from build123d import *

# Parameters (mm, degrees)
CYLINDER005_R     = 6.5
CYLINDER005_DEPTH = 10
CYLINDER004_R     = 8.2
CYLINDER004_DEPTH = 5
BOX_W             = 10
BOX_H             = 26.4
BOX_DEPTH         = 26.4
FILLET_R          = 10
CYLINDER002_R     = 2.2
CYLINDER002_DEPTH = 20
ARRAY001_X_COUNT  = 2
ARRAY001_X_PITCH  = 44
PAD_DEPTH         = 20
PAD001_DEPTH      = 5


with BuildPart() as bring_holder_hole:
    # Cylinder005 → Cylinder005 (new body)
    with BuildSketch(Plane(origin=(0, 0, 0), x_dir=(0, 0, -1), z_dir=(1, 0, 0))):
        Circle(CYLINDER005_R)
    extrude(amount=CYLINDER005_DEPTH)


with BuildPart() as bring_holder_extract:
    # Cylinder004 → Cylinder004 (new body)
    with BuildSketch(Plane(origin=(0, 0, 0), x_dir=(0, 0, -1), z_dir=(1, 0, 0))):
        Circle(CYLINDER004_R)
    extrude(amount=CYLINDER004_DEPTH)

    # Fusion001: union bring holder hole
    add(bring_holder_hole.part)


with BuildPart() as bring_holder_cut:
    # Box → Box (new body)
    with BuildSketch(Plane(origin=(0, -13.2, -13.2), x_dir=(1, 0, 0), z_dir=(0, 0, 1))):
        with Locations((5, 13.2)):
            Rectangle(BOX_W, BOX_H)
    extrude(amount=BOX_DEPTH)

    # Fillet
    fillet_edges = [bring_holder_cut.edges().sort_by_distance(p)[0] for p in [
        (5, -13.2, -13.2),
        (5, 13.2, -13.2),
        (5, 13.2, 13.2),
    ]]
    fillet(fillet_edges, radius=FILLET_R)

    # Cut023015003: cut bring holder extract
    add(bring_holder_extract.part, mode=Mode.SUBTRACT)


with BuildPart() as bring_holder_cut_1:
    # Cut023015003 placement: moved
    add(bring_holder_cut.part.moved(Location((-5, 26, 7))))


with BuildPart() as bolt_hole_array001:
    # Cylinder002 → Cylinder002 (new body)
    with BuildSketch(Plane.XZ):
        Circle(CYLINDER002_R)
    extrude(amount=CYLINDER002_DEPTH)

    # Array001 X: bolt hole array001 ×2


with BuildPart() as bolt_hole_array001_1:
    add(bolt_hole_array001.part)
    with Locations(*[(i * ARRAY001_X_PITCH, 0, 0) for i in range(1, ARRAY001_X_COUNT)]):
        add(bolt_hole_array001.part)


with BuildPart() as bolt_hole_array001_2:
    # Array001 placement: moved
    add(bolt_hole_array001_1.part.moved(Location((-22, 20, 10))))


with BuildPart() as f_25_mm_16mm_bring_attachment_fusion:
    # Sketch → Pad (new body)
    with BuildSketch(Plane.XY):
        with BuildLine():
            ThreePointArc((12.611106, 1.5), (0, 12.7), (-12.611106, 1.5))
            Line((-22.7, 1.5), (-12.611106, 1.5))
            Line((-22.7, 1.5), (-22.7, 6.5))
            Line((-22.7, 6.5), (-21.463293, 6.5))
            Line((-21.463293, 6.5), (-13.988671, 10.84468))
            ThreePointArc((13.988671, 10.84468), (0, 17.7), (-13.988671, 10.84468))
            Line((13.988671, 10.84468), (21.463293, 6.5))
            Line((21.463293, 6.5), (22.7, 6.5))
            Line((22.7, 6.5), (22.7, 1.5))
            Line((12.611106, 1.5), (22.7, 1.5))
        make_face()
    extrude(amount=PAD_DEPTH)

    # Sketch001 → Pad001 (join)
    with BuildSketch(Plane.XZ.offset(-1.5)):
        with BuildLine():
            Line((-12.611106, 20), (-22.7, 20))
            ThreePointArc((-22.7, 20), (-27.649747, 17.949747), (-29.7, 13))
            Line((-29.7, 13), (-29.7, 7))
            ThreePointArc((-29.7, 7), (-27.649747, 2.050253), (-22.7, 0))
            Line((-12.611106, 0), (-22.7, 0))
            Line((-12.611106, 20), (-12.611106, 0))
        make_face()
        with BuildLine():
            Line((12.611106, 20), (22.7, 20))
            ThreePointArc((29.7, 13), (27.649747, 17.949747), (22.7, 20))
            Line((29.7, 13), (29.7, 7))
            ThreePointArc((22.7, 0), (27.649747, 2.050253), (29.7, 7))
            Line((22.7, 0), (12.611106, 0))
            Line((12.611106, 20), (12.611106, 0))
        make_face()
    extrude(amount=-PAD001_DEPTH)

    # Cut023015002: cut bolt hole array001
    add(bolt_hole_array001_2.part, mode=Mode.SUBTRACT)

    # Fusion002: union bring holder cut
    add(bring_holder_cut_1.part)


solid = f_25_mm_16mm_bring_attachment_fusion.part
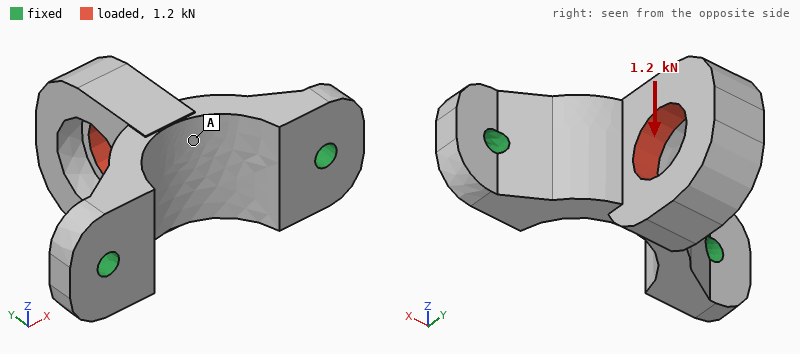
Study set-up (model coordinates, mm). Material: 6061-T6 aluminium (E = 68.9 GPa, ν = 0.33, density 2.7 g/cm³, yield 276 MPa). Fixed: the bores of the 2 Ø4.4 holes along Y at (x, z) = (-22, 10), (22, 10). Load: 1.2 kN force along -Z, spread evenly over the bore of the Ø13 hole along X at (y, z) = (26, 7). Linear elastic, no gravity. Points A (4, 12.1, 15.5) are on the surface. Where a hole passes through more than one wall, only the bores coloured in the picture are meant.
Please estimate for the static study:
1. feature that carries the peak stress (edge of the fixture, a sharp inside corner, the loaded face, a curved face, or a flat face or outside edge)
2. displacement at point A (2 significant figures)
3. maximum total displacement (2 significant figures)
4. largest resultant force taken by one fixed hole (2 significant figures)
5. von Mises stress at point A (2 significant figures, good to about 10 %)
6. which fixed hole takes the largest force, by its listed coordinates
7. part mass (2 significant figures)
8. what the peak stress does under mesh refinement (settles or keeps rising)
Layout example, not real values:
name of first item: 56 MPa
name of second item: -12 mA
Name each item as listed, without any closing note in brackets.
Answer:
feature that carries the peak stress: edge of the fixture
displacement at point A: 0.045 mm
maximum total displacement: 0.19 mm
largest resultant force taken by one fixed hole: 670 N
von Mises stress at point A: 30 MPa
which fixed hole takes the largest force, by its listed coordinates: (22, 10)
part mass: 29 g
what the peak stress does under mesh refinement: keeps rising
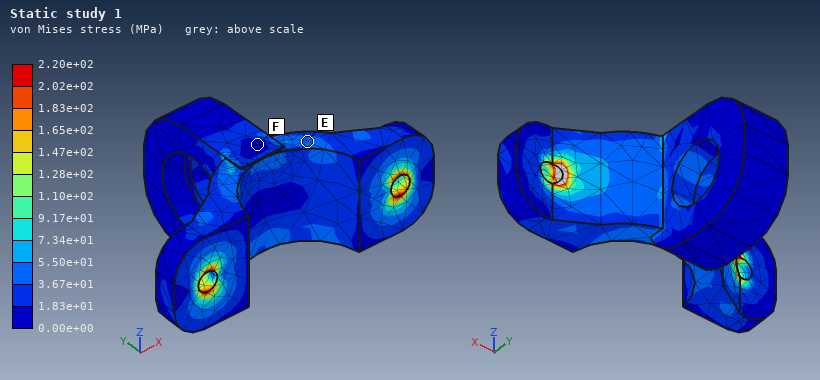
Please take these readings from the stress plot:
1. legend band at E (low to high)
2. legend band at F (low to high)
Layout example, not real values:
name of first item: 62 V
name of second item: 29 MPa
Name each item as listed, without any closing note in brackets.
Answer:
legend band at E: 3.67e+01 to 5.50e+01 MPa
legend band at F: 0.00e+00 to 1.83e+01 MPa
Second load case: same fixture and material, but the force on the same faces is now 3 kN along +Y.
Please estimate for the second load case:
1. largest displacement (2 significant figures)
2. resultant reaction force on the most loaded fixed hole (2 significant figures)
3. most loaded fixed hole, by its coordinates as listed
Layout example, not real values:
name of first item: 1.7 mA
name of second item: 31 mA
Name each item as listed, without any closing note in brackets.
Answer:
largest displacement: 91 µm
resultant reaction force on the most loaded fixed hole: 2.6 kN
most loaded fixed hole, by its coordinates as listed: (22, 10)
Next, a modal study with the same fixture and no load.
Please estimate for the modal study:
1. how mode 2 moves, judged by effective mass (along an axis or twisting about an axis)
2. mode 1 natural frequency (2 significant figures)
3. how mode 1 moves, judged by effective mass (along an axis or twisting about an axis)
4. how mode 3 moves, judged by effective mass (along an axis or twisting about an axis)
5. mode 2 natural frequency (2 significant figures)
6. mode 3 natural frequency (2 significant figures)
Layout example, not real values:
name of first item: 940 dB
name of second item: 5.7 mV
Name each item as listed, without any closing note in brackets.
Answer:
how mode 2 moves, judged by effective mass: along X
mode 1 natural frequency: 4000 Hz
how mode 1 moves, judged by effective mass: along Z
how mode 3 moves, judged by effective mass: along Y
mode 2 natural frequency: 7100 Hz
mode 3 natural frequency: 15 kHz
